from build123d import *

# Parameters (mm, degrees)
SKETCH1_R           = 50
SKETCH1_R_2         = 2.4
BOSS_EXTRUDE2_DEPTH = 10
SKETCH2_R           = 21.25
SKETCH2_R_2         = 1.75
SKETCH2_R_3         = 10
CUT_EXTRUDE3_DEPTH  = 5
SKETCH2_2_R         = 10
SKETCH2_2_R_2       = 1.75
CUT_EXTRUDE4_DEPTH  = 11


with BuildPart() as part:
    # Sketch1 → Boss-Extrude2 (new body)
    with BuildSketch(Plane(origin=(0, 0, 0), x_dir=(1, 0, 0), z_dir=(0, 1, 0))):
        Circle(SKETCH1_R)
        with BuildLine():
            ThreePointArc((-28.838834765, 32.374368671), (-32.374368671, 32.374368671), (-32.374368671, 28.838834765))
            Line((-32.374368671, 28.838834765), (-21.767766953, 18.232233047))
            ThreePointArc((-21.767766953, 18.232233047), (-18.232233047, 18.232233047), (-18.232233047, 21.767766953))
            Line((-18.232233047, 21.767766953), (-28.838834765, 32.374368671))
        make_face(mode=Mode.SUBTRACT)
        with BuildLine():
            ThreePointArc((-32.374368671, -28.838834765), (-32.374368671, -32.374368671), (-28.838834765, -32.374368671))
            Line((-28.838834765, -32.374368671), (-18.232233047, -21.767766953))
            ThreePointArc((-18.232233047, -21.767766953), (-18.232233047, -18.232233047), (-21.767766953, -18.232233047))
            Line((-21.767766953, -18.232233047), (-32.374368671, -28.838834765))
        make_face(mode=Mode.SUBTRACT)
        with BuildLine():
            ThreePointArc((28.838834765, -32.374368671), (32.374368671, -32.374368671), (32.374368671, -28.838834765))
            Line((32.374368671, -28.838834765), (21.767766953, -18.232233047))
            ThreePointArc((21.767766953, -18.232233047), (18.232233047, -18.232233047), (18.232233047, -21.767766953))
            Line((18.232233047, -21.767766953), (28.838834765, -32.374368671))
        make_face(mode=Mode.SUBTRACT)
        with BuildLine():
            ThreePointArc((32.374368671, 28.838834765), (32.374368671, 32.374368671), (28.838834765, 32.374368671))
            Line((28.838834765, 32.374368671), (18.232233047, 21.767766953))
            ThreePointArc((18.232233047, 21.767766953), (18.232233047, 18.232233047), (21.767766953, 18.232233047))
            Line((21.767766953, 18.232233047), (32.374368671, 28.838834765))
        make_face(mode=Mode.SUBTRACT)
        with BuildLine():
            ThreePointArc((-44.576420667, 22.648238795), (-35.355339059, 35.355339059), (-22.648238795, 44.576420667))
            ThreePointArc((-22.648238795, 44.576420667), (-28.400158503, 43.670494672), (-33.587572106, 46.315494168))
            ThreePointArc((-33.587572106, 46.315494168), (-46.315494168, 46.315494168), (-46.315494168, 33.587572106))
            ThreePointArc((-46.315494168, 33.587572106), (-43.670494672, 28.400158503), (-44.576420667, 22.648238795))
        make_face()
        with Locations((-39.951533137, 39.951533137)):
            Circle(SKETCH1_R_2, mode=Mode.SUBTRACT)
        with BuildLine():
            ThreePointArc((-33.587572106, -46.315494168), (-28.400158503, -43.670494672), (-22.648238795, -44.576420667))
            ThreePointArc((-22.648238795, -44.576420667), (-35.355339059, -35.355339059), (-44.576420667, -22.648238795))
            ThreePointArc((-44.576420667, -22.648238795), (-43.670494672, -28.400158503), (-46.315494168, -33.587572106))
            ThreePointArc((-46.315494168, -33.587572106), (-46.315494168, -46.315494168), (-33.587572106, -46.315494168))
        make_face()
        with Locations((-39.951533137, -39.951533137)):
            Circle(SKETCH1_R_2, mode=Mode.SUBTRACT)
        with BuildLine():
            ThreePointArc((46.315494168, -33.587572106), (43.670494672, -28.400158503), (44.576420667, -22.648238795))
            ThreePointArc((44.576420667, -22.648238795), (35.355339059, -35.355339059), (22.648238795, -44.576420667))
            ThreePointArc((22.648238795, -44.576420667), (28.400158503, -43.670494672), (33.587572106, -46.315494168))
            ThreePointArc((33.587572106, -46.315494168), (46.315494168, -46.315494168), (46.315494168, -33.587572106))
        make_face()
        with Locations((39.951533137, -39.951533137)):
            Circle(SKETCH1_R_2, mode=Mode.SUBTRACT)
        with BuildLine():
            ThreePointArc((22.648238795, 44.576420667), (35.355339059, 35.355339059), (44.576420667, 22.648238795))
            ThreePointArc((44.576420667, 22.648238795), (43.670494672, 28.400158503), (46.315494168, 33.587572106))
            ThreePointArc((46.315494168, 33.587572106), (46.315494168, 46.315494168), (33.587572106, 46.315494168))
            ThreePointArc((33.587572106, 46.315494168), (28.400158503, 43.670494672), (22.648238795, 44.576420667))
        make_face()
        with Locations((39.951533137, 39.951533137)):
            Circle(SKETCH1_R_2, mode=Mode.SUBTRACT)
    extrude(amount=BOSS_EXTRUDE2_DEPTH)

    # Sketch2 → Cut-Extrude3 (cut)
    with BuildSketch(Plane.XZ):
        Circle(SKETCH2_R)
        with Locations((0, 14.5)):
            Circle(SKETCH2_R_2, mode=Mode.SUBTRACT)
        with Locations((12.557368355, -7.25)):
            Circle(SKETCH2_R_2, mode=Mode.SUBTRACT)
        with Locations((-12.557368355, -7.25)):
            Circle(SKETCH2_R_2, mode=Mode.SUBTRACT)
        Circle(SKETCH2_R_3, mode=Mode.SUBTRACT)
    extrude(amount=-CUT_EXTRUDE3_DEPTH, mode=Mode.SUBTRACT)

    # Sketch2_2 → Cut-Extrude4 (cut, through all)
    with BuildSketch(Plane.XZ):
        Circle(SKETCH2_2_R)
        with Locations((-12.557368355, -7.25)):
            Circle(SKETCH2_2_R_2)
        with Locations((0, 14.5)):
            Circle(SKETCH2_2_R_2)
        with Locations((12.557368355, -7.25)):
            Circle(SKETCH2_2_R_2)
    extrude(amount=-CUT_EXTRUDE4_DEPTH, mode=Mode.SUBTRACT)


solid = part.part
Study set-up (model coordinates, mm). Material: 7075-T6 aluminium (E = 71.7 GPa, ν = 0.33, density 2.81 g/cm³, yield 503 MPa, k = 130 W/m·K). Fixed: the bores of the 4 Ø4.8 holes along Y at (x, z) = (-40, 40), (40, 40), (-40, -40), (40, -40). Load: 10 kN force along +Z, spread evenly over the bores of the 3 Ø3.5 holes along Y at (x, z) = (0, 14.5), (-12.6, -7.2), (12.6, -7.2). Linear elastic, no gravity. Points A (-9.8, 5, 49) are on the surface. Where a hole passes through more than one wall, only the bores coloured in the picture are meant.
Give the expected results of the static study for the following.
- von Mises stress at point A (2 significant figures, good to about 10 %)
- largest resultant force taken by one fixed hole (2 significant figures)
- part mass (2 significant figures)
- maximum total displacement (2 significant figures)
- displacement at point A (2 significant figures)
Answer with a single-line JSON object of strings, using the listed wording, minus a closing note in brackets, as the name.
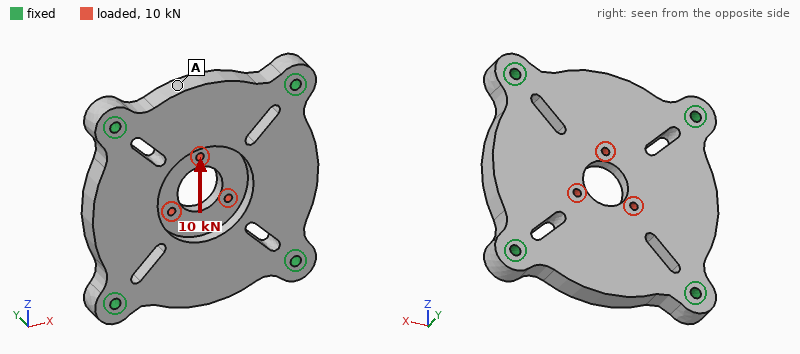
{"von Mises stress at point A": "9.5 MPa", "largest resultant force taken by one fixed hole": "2.9 kN", "part mass": "210 g", "maximum total displacement": "24 µm", "displacement at point A": "13 µm"}
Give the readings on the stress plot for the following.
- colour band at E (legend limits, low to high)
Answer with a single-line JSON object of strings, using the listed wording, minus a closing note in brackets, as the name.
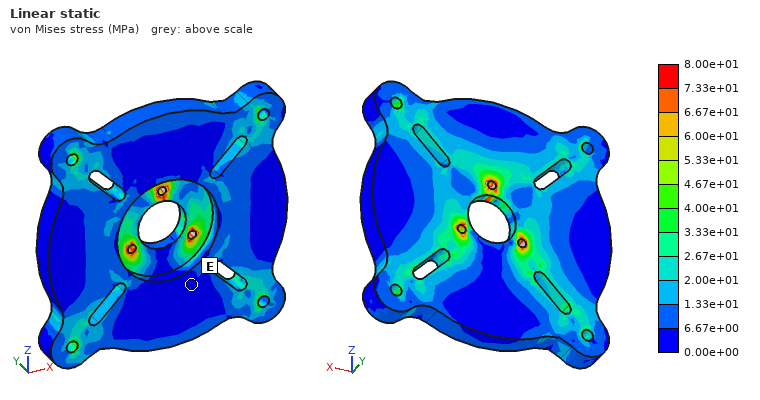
{"colour band at E": "0.00e+00 to 6.67e+00 MPa"}
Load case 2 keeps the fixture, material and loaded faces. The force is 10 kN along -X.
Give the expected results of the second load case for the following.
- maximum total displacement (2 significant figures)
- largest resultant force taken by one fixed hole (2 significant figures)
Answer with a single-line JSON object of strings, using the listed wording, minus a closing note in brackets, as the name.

{"maximum total displacement": "22 µm", "largest resultant force taken by one fixed hole": "3.0 kN"}
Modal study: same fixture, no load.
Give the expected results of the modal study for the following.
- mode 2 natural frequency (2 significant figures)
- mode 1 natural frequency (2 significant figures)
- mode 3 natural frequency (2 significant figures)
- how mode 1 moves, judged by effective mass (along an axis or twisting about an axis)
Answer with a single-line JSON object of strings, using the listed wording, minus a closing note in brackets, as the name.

{"mode 2 natural frequency": "6900 Hz", "mode 1 natural frequency": "4800 Hz", "mode 3 natural frequency": "6900 Hz", "how mode 1 moves, judged by effective mass": "along Y"}
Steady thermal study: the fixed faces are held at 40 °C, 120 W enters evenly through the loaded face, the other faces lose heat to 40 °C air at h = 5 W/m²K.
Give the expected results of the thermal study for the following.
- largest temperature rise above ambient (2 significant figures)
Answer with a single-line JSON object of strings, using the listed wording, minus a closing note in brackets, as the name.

{"largest temperature rise above ambient": "58 K"}
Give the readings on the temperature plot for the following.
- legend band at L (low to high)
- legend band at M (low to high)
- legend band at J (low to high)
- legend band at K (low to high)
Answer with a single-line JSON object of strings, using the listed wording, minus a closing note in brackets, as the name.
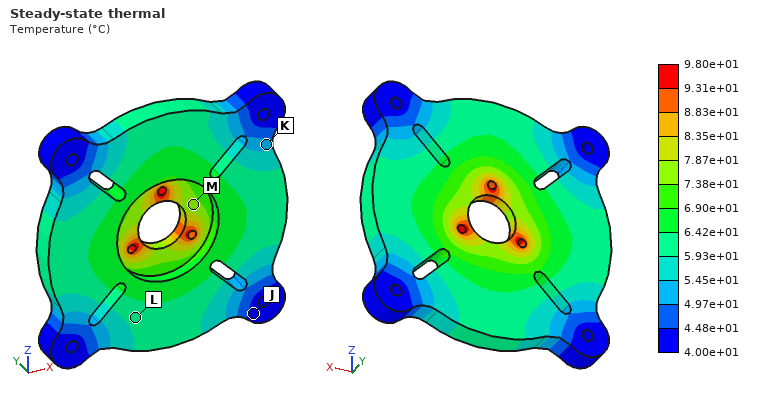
{"legend band at L": "5.93e+01 to 6.42e+01 °C", "legend band at M": "7.38e+01 to 7.87e+01 °C", "legend band at J": "4.00e+01 to 4.48e+01 °C", "legend band at K": "4.97e+01 to 5.45e+01 °C"}
